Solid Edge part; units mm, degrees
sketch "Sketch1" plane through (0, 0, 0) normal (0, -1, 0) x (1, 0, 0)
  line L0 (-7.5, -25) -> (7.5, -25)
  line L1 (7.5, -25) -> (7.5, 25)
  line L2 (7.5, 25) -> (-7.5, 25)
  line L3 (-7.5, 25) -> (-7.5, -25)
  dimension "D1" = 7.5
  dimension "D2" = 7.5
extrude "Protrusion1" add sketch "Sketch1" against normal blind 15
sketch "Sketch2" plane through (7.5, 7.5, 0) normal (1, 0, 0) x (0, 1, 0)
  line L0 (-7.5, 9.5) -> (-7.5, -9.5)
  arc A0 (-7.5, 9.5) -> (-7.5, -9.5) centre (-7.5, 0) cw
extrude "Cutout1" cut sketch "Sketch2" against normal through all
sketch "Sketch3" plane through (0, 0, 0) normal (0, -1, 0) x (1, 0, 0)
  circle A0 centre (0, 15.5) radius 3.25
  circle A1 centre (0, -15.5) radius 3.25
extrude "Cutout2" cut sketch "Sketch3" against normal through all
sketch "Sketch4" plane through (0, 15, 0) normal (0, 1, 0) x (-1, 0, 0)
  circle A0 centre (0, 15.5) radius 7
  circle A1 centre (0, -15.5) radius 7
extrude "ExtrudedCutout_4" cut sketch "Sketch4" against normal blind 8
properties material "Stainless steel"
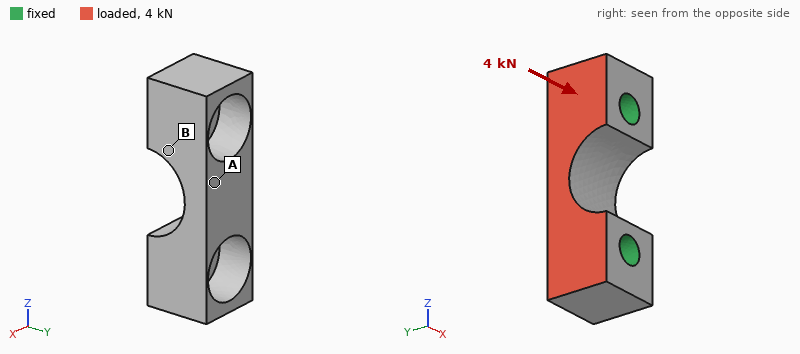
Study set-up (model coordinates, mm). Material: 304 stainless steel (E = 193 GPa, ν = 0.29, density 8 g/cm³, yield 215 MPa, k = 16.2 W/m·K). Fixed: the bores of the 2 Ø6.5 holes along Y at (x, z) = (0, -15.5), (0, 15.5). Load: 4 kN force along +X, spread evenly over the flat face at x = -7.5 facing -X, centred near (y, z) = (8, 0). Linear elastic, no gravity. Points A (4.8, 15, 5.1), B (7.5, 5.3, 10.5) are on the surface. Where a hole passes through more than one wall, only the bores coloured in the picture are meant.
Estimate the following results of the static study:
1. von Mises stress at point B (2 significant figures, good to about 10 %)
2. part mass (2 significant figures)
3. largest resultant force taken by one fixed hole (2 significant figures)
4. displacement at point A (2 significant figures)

32 MPa
50 g
2.0 kN
5.2 µm
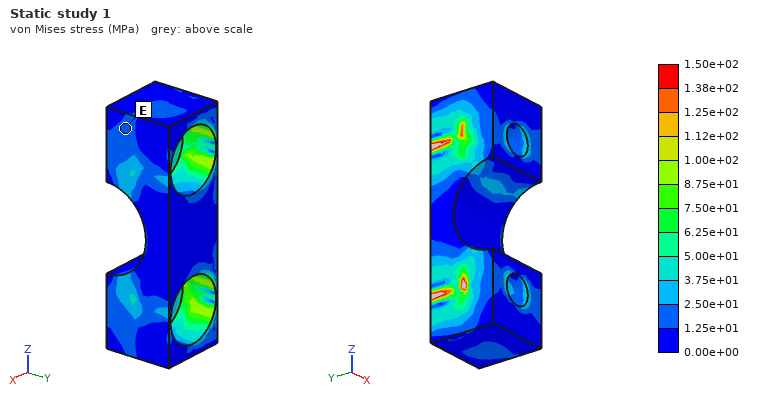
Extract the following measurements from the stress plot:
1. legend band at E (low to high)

1.25e+01 to 2.50e+01 MPa
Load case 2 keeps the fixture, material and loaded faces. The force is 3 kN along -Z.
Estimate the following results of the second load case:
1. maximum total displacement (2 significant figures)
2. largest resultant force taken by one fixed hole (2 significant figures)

5.5 µm
1.6 kN
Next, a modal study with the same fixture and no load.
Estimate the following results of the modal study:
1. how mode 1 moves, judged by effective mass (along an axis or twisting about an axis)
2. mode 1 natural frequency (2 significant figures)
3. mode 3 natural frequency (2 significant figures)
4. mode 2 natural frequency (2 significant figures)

along X
21 kHz
30 kHz
30 kHz
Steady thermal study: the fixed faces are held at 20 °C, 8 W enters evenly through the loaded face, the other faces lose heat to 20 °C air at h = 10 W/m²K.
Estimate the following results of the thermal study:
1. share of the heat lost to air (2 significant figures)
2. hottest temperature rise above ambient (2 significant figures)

3.1 %
25 K
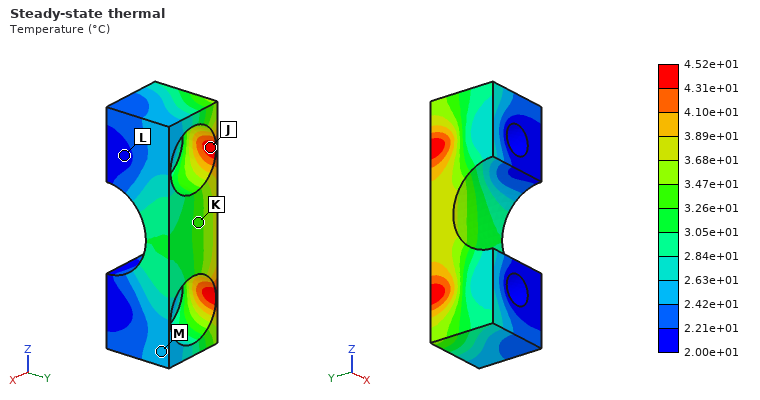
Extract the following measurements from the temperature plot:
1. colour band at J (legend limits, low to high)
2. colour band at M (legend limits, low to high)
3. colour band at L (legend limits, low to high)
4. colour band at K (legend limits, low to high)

4.31e+01 to 4.52e+01 °C
2.42e+01 to 2.63e+01 °C
2.00e+01 to 2.21e+01 °C
3.26e+01 to 3.47e+01 °C
